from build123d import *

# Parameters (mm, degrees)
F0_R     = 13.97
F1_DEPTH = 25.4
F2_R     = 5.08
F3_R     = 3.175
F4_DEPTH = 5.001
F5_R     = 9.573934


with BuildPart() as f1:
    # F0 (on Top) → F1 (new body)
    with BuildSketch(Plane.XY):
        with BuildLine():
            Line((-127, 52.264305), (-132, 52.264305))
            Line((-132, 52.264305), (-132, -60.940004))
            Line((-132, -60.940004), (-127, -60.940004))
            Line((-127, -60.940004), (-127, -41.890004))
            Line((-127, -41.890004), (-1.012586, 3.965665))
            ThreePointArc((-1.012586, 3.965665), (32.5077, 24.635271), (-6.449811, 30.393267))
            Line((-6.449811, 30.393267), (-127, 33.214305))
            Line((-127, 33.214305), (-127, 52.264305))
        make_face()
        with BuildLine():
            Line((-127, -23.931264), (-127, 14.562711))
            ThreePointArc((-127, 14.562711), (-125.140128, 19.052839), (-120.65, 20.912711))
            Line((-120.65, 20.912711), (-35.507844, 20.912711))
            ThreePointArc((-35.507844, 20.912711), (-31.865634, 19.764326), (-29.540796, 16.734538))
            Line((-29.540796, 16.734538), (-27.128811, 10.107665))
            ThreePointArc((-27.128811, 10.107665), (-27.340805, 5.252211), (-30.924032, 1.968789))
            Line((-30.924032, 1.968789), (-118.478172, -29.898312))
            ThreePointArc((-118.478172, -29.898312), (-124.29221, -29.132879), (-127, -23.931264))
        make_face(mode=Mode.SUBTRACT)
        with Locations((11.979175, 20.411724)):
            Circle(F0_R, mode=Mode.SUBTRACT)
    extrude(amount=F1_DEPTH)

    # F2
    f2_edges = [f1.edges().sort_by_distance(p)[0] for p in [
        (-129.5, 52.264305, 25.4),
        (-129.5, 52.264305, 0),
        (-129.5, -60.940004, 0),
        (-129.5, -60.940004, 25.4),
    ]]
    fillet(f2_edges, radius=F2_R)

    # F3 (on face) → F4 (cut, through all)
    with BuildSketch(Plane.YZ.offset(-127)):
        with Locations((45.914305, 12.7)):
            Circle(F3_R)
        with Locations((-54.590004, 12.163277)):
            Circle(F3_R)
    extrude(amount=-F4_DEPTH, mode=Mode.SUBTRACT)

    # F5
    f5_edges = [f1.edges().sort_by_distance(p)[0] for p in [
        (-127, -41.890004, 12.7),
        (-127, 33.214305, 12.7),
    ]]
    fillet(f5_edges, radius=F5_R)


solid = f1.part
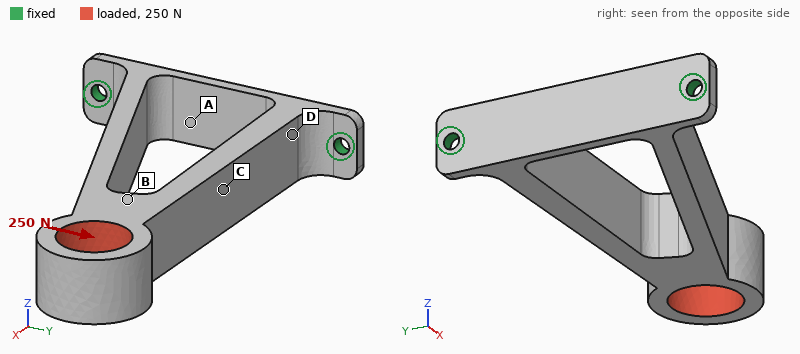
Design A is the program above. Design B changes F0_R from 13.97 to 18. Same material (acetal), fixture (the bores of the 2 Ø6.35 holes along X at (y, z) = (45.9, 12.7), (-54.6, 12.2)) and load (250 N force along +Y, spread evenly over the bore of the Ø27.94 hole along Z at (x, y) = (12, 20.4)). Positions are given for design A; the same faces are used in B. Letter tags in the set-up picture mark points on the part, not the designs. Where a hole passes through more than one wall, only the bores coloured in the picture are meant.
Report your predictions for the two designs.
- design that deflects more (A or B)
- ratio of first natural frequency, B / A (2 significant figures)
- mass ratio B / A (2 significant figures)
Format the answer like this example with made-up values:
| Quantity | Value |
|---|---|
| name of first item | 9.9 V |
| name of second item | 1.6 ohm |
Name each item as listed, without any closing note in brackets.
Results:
| Quantity | Value |
|---|---|
| design that deflects more | B |
| ratio of first natural frequency, B / A | 1.2 |
| mass ratio B / A | 0.90 |
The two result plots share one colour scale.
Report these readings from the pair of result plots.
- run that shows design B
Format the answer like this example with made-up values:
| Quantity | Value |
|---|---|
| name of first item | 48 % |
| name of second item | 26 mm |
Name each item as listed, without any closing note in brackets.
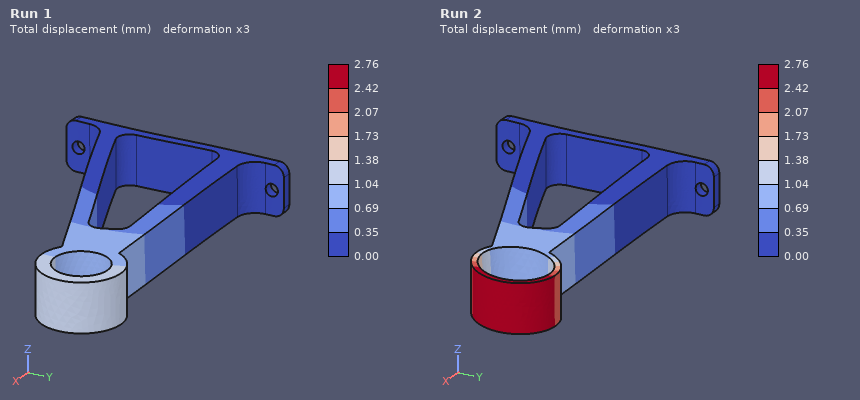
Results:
| Quantity | Value |
|---|---|
| run that shows design B | Run 2 |
